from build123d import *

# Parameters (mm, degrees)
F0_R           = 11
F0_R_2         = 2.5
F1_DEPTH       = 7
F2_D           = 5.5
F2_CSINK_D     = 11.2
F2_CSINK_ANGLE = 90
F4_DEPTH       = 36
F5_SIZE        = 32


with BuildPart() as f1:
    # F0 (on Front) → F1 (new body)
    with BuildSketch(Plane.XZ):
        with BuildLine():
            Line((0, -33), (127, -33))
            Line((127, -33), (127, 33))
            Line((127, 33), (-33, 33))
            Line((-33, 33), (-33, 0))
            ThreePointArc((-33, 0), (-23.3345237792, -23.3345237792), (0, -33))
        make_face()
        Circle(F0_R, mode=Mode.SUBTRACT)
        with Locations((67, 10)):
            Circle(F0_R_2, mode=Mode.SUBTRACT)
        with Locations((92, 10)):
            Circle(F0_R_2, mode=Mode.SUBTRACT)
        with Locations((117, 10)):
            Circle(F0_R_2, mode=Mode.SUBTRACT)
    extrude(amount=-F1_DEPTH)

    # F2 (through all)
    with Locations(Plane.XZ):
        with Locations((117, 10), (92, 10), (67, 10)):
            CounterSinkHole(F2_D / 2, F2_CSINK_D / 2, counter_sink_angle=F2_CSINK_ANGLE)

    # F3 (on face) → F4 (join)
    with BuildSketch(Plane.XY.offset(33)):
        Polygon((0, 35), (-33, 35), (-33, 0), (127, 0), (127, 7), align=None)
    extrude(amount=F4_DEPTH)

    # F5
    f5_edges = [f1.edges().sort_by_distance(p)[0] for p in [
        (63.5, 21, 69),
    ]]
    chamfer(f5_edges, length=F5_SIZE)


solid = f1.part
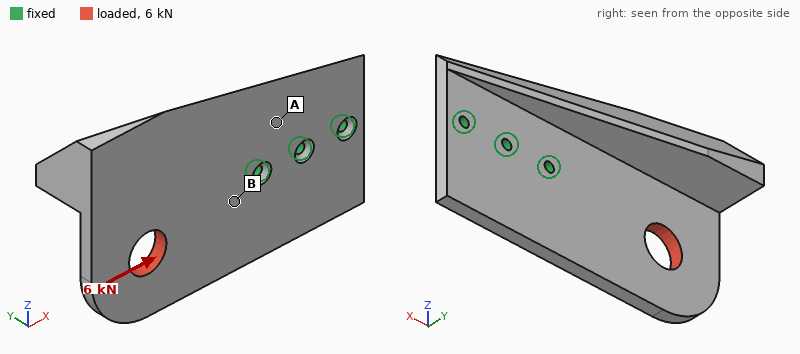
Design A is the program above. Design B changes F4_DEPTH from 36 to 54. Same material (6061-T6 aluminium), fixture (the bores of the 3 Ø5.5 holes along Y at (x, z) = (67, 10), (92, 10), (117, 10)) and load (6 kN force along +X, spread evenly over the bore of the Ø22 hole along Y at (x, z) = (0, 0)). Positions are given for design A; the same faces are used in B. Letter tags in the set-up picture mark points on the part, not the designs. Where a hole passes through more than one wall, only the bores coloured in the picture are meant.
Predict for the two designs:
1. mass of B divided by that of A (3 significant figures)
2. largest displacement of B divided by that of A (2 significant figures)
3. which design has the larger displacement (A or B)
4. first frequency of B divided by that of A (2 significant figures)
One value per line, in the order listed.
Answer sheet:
1.50
0.84
A
0.78
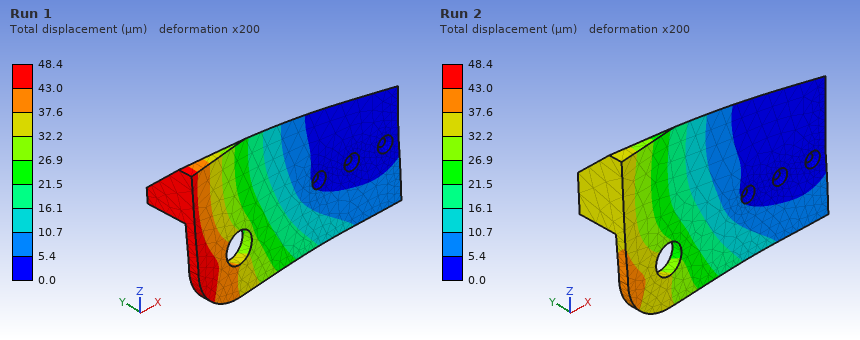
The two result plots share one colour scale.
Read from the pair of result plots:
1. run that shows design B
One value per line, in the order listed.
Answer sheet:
Run 2
